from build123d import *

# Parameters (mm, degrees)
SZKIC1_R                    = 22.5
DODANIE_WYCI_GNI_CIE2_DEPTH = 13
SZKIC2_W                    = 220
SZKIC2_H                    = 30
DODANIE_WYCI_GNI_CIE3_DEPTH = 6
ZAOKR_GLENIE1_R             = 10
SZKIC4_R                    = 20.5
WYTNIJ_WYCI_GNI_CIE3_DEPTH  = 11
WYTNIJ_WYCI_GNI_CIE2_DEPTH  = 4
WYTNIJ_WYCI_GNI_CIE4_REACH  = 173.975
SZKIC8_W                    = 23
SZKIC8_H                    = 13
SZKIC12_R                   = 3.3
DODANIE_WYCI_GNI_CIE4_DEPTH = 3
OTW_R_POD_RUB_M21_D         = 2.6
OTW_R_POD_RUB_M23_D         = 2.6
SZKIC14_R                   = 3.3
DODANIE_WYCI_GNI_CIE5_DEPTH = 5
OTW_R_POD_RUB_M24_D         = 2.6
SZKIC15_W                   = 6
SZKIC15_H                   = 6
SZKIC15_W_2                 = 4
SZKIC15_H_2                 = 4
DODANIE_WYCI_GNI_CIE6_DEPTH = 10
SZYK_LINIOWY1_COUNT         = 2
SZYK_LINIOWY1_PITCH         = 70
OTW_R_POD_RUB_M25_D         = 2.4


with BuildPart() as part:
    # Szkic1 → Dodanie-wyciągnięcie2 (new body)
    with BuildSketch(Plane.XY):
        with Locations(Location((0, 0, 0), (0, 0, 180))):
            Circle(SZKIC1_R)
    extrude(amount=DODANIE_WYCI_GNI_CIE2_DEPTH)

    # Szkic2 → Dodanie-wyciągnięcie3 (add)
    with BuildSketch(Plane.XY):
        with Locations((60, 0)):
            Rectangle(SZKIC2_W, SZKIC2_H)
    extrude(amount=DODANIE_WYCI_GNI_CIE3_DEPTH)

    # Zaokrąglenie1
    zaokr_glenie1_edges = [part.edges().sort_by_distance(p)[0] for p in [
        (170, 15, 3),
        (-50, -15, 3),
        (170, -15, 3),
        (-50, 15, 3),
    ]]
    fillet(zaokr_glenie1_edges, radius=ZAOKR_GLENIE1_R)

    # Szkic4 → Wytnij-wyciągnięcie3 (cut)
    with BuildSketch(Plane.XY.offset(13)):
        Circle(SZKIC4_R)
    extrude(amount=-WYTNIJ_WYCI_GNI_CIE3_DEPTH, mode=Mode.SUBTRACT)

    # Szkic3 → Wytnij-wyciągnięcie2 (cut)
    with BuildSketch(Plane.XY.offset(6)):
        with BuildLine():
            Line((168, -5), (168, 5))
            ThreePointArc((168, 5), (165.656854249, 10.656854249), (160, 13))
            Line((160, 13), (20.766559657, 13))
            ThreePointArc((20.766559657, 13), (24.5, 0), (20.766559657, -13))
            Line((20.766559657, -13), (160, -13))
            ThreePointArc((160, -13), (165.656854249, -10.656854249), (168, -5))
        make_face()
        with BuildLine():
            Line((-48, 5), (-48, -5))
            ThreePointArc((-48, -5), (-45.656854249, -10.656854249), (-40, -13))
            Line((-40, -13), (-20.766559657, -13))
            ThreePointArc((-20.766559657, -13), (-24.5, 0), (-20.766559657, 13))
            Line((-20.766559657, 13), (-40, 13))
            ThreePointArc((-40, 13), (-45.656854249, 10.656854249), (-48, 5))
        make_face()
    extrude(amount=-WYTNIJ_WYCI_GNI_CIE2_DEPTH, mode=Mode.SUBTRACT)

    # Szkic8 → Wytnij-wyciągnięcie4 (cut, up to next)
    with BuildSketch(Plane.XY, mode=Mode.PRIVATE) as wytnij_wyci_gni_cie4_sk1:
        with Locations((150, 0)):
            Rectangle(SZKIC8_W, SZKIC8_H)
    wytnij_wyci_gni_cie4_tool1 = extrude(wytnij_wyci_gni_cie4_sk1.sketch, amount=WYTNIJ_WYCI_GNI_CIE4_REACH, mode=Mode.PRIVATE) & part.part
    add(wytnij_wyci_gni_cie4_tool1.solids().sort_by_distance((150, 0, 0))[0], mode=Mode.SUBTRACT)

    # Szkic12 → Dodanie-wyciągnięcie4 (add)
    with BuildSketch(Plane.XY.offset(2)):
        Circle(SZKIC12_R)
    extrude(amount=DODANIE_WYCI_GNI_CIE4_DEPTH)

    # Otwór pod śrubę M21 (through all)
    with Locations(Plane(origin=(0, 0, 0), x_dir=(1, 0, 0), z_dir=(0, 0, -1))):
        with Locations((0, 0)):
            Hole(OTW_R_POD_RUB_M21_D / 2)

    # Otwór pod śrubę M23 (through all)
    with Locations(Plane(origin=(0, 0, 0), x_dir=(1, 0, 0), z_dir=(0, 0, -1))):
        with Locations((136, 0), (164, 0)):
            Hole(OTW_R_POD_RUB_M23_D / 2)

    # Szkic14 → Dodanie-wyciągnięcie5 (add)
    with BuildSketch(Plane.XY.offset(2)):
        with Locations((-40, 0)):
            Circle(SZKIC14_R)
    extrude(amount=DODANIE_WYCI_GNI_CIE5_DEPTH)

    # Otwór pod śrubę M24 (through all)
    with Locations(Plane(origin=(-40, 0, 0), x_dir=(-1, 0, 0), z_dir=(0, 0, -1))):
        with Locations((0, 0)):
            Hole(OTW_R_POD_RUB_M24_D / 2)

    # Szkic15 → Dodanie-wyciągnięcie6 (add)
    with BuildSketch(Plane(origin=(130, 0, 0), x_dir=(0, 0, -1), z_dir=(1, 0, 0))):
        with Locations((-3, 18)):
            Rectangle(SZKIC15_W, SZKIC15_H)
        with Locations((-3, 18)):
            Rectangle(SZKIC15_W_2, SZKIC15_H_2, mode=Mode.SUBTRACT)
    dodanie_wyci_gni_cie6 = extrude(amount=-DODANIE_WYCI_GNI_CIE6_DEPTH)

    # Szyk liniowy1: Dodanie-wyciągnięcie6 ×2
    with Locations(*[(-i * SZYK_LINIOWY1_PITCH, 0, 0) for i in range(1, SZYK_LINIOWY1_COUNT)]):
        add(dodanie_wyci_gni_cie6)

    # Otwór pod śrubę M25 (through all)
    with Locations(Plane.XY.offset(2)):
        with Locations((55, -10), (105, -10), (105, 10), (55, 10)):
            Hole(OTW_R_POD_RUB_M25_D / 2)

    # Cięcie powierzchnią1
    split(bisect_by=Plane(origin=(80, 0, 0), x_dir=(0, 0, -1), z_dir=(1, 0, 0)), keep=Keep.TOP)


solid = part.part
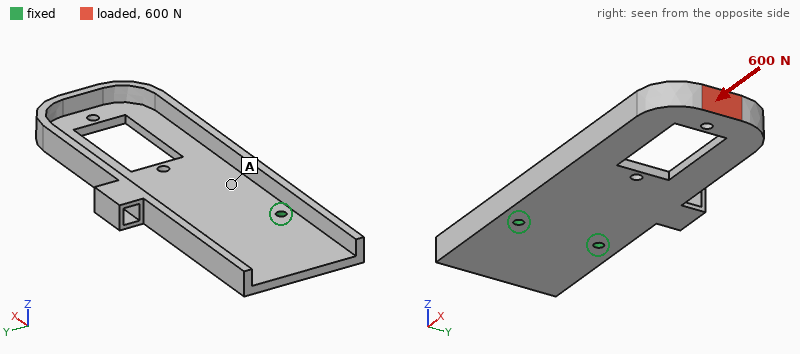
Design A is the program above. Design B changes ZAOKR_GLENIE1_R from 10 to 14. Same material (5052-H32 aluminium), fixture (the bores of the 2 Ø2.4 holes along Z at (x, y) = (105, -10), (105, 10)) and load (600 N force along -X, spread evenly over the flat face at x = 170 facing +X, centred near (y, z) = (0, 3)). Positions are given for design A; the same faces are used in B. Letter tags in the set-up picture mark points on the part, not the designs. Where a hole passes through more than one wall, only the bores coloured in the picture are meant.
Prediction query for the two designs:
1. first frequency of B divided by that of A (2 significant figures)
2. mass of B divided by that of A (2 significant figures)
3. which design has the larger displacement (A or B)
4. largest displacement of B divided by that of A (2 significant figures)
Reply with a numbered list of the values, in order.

1. 1.1
2. 0.96
3. B
4. 1.2
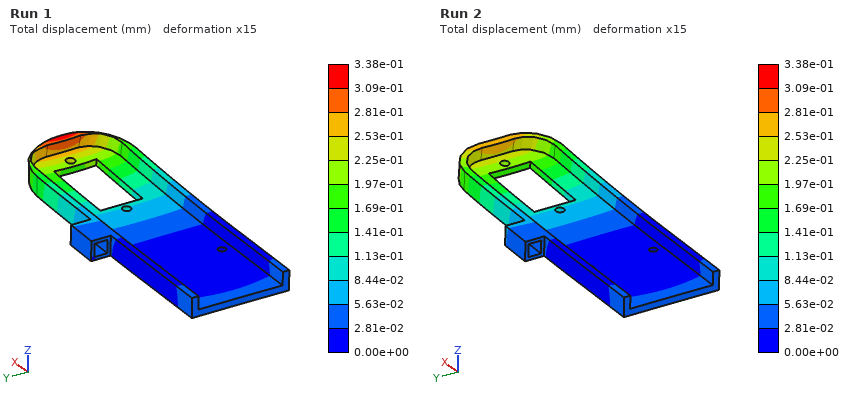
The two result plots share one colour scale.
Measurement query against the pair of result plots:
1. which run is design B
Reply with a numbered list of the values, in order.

1. Run 1
